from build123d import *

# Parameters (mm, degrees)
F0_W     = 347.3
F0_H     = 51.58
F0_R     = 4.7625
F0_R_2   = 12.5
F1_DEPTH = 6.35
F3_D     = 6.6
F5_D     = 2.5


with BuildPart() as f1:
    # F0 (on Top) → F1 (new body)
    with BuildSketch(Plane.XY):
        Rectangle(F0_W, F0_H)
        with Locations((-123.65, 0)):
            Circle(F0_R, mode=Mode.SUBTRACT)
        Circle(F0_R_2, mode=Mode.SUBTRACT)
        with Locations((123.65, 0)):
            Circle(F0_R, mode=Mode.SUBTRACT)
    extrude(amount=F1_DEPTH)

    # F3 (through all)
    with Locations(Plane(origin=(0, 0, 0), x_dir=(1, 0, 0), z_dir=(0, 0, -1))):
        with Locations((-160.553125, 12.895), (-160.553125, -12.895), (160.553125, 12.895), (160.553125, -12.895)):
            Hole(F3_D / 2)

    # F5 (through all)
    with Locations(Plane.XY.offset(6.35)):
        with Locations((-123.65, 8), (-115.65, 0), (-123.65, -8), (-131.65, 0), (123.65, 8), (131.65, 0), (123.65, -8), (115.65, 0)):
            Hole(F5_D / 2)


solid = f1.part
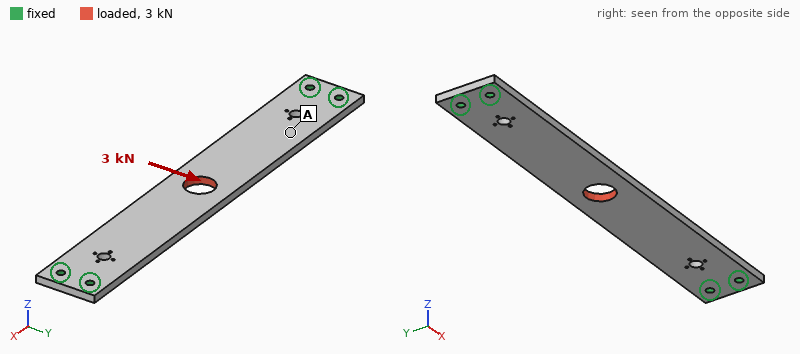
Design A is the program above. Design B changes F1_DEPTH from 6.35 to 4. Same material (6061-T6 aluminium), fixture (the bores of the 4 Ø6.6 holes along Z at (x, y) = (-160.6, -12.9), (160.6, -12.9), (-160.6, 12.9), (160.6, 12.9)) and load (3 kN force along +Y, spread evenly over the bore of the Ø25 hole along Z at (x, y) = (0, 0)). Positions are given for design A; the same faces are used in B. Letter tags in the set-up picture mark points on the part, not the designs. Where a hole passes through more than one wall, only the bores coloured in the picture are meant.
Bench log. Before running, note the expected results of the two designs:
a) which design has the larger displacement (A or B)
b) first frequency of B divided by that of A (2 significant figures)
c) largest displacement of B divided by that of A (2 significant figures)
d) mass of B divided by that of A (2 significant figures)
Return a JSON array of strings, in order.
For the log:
["B", "0.64", "1.6", "0.63"]
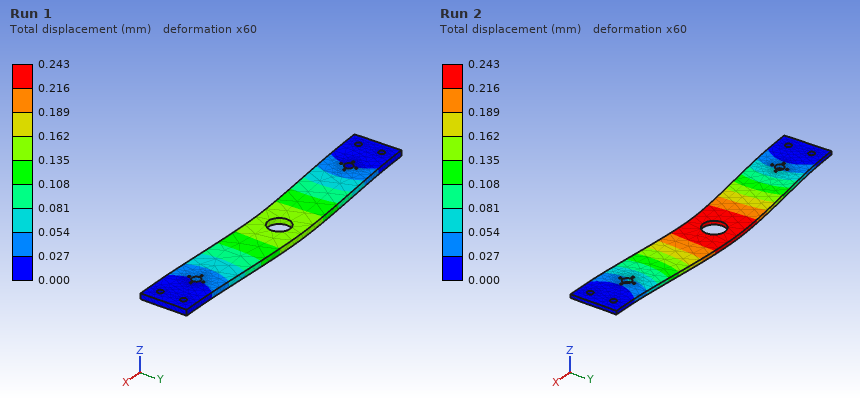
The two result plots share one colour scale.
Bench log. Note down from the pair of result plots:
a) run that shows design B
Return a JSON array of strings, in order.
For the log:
["Run 2"]
